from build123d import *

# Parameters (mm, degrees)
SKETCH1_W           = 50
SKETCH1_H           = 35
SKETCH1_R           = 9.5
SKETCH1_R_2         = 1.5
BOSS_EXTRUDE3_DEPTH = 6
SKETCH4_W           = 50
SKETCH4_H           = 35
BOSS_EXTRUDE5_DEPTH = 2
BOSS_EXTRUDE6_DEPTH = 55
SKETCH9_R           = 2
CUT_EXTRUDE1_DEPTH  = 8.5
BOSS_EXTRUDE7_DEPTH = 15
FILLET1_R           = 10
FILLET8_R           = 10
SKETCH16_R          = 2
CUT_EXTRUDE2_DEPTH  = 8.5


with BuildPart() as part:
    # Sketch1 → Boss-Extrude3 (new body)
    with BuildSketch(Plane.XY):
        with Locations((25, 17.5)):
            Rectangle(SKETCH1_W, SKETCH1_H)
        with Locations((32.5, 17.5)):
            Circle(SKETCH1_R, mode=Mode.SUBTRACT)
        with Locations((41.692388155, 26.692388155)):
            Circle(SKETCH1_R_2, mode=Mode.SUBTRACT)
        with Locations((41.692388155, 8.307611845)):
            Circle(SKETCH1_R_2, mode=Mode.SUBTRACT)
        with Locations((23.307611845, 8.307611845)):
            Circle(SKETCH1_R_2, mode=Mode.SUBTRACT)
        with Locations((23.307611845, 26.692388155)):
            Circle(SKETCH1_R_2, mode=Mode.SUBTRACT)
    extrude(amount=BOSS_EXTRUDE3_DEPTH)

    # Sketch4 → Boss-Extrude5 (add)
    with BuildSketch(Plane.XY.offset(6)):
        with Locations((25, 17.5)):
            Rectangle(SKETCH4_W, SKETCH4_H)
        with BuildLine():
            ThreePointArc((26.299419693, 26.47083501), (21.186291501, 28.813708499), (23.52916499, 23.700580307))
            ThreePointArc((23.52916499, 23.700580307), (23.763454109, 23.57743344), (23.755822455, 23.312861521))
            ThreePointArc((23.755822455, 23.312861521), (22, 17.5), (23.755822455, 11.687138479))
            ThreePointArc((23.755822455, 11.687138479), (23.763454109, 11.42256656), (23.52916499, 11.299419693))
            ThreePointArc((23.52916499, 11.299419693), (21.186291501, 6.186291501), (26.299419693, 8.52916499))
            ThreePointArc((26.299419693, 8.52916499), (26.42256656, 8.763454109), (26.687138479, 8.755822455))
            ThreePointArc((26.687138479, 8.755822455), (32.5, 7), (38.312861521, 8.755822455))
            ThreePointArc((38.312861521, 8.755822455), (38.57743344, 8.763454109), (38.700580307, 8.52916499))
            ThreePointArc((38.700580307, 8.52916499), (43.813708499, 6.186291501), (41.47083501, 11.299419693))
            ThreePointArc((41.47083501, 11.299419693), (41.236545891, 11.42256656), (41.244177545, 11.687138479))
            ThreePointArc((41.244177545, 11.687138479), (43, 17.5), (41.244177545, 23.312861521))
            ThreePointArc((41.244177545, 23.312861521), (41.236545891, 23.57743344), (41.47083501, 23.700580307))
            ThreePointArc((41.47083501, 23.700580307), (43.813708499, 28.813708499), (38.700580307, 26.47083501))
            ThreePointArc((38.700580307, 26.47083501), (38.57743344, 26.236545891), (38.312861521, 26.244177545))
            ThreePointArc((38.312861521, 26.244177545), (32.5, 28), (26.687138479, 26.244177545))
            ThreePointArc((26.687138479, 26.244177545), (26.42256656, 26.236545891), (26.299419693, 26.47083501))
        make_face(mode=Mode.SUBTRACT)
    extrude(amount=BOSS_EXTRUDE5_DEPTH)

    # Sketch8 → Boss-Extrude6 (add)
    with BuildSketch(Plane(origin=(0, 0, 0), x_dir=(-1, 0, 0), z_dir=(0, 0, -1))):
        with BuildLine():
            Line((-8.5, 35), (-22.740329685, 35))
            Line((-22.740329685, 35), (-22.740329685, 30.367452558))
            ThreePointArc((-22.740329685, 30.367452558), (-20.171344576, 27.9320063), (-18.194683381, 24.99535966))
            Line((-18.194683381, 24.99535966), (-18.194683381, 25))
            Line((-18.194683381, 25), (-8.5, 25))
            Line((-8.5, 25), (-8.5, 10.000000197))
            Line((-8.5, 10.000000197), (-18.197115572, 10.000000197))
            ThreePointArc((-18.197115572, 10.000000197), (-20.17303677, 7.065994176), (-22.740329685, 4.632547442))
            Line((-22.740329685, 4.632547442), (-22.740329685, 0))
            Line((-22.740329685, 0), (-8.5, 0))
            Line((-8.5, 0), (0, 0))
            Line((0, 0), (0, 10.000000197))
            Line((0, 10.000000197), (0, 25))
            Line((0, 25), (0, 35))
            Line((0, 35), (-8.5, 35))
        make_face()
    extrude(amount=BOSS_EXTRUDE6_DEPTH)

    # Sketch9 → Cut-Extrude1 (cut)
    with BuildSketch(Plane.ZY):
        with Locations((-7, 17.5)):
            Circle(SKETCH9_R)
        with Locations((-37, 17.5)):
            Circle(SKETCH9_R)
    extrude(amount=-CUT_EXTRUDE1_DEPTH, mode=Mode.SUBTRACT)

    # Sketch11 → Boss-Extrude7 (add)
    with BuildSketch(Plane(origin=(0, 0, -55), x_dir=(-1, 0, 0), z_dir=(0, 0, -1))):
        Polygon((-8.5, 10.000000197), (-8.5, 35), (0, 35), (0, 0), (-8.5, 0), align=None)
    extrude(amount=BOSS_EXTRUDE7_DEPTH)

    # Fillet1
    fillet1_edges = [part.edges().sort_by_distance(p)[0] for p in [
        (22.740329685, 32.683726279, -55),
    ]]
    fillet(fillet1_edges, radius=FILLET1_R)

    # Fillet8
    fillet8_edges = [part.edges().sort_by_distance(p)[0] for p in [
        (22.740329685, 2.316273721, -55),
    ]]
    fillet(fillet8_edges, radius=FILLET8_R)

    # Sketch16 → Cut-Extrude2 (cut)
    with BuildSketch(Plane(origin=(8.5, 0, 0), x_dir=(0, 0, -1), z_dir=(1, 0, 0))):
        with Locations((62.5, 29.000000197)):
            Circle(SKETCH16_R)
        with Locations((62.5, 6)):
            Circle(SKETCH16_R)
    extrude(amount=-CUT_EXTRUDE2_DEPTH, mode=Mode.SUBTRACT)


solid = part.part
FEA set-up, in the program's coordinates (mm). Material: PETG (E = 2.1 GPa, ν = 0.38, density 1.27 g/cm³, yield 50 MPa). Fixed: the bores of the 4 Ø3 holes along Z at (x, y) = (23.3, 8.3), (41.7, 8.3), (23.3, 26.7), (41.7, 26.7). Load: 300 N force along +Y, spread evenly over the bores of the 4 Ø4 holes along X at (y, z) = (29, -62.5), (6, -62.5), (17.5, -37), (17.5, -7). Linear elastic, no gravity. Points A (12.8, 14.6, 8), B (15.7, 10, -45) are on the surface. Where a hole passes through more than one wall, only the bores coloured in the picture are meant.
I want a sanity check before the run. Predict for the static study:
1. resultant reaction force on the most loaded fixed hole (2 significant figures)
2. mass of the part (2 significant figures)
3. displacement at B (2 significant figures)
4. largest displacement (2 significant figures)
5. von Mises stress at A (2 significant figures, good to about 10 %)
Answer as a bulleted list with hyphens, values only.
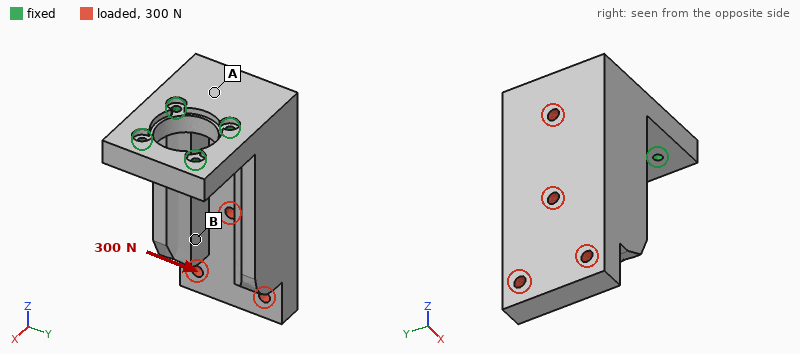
- 590 N
- 58 g
- 0.81 mm
- 1.2 mm
- 5.1 MPa
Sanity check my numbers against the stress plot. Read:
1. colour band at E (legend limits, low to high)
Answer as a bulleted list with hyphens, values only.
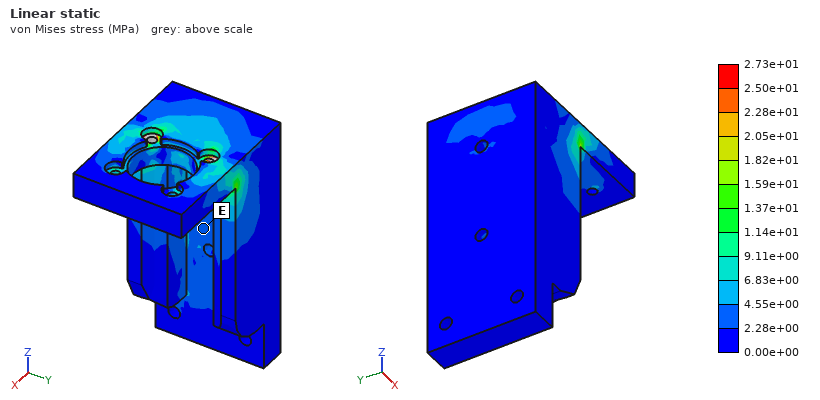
- 2.28e+00 to 4.55e+00 MPa
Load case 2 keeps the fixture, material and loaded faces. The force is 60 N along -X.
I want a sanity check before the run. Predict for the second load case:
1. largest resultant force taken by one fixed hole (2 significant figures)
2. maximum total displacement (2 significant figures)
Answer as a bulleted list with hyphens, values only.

- 49 N
- 0.93 mm
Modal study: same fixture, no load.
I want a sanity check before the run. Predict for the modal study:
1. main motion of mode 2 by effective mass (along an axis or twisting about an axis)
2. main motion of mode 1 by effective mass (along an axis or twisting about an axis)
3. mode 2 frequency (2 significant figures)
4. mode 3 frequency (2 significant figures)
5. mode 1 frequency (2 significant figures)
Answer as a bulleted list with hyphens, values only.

- along Y
- along X
- 530 Hz
- 1500 Hz
- 280 Hz
